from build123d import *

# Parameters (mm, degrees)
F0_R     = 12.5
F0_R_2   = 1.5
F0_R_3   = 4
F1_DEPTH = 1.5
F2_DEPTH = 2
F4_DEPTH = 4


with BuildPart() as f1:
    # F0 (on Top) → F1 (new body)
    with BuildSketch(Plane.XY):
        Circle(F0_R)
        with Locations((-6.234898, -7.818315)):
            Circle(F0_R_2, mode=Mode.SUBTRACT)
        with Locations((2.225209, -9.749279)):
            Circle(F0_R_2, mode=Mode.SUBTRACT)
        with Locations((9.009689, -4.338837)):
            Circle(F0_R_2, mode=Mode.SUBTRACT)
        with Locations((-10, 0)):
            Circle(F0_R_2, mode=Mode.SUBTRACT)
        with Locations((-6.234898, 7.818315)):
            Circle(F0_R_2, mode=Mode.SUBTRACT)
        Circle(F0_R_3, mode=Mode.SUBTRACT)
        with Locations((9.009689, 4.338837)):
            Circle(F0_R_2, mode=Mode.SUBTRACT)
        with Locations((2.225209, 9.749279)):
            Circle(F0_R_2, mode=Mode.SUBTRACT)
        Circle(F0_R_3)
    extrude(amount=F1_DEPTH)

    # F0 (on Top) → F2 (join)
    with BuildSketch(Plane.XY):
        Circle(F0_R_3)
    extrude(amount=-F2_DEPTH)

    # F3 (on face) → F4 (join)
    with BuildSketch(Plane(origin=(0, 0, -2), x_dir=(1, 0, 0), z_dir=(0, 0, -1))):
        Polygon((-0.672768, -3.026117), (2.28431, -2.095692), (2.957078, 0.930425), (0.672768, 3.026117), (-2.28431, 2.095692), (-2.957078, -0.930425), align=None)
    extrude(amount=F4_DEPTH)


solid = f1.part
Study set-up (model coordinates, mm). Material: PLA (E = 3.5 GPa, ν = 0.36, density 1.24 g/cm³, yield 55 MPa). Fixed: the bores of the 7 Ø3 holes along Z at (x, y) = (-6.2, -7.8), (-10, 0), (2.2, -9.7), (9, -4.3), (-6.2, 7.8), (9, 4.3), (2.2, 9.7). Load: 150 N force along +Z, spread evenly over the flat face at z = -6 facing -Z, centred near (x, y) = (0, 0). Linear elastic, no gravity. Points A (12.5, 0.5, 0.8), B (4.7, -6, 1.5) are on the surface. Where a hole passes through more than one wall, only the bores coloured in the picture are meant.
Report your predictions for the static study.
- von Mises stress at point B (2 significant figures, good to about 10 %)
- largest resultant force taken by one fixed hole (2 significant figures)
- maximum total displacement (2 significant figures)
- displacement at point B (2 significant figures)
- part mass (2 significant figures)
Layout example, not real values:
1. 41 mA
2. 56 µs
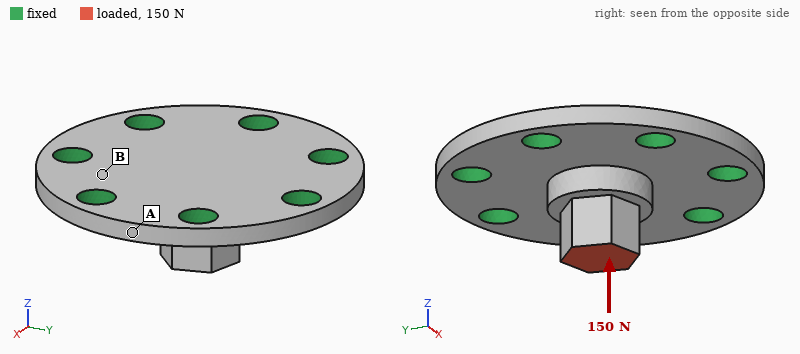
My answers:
1. 10 MPa
2. 24 N
3. 82 µm
4. 17 µm
5. 1.1 g
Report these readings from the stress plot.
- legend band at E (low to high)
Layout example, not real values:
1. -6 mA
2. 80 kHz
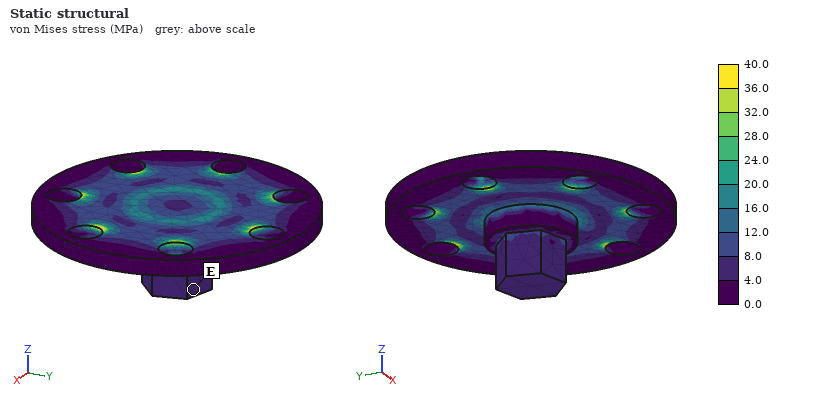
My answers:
1. 4.0 to 8.0 MPa
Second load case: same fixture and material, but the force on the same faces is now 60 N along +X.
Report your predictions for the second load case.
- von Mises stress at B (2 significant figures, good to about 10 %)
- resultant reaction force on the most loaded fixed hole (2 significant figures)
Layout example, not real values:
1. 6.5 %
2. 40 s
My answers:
1. 4.0 MPa
2. 23 N
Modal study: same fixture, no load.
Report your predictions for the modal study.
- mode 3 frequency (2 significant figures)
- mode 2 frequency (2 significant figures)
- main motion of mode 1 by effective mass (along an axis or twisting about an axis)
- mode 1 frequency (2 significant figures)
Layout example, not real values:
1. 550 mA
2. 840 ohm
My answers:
1. 14 kHz
2. 14 kHz
3. along Z
4. 11 kHz
